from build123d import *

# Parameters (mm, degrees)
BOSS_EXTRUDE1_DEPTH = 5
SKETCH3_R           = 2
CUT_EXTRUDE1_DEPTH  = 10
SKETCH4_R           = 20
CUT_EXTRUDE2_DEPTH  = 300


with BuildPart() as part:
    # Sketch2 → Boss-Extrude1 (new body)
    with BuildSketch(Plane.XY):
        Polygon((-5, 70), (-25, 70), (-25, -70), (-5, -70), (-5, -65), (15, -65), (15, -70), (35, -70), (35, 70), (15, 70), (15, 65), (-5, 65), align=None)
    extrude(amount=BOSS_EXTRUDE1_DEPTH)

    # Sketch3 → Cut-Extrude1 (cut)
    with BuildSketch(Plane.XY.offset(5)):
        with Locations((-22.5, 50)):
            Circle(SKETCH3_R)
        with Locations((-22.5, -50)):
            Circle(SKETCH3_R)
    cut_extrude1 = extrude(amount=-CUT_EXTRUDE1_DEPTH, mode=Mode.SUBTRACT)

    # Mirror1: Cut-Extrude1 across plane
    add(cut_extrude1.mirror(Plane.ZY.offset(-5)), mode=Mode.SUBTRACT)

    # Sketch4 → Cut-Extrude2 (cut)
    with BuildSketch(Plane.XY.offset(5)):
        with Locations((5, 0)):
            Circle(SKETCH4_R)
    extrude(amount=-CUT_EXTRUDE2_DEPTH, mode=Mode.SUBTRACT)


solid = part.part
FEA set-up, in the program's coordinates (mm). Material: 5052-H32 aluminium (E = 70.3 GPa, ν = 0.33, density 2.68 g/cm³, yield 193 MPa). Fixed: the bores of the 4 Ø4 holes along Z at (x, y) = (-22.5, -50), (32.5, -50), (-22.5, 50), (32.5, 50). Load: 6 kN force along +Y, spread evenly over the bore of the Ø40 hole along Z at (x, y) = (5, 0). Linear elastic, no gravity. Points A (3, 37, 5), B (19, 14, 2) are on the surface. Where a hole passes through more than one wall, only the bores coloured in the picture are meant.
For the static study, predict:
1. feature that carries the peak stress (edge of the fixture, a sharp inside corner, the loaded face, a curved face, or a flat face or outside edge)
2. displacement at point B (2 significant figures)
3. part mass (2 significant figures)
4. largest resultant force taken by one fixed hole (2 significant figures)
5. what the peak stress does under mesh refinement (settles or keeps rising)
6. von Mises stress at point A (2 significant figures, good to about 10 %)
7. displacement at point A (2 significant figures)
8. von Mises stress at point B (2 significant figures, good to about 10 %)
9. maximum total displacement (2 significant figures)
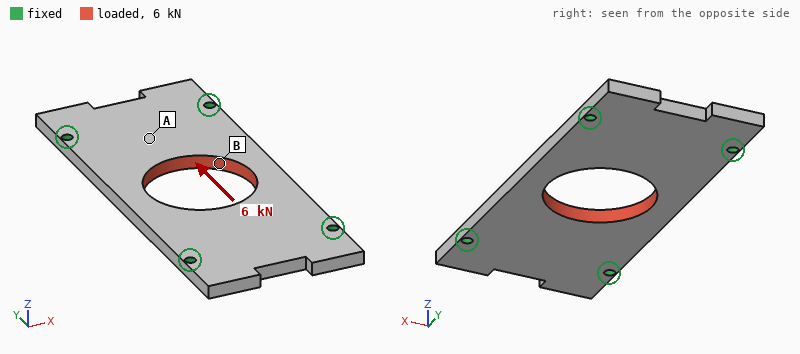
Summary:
edge of the fixture
8.9 µm
92 g
1.5 kN
keeps rising
4.9 MPa
7.0 µm
13 MPa
10 µm
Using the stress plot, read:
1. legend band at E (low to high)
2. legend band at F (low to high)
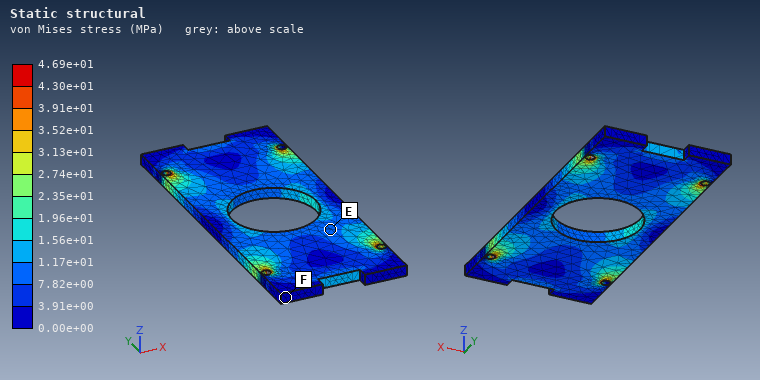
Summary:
7.82e+00 to 1.17e+01 MPa
0.00e+00 to 3.91e+00 MPa
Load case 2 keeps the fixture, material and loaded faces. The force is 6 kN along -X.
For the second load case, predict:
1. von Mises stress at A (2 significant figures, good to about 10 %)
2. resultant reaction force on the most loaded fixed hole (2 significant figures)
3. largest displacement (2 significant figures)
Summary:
24 MPa
1.9 kN
32 µm
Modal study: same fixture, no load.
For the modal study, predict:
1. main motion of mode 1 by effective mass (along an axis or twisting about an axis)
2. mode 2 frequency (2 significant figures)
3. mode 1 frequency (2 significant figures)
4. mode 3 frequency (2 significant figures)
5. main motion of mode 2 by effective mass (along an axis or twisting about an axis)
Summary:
along Z
3700 Hz
2400 Hz
5100 Hz
twisting about Y
